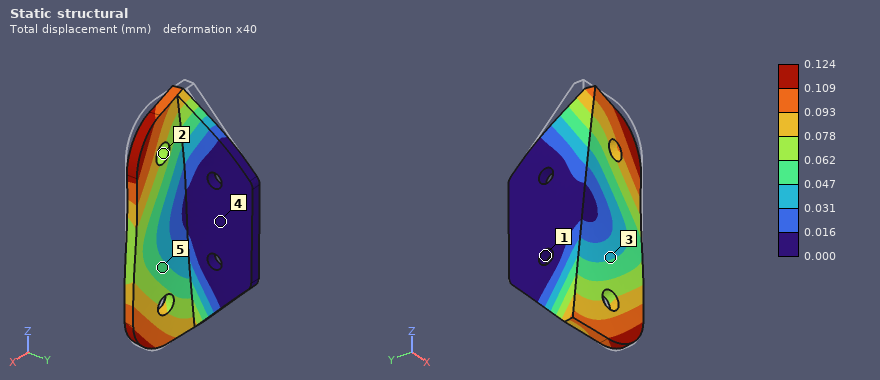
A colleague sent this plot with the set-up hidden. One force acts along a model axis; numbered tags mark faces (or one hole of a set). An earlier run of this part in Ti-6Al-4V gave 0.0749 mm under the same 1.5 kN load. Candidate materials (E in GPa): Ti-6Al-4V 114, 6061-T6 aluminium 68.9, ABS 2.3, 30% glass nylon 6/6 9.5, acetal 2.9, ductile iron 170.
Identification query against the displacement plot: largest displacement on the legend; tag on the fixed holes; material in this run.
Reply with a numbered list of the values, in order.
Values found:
1. 0.124 mm
2. 1
3. 6061-T6 aluminium
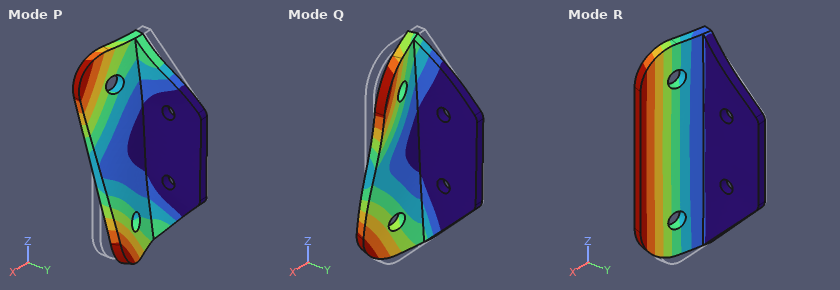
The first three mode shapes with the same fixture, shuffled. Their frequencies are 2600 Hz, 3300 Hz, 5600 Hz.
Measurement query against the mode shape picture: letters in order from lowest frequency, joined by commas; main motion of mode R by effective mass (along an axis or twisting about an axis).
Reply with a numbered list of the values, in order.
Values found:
1. R, Q, P
2. along Y
